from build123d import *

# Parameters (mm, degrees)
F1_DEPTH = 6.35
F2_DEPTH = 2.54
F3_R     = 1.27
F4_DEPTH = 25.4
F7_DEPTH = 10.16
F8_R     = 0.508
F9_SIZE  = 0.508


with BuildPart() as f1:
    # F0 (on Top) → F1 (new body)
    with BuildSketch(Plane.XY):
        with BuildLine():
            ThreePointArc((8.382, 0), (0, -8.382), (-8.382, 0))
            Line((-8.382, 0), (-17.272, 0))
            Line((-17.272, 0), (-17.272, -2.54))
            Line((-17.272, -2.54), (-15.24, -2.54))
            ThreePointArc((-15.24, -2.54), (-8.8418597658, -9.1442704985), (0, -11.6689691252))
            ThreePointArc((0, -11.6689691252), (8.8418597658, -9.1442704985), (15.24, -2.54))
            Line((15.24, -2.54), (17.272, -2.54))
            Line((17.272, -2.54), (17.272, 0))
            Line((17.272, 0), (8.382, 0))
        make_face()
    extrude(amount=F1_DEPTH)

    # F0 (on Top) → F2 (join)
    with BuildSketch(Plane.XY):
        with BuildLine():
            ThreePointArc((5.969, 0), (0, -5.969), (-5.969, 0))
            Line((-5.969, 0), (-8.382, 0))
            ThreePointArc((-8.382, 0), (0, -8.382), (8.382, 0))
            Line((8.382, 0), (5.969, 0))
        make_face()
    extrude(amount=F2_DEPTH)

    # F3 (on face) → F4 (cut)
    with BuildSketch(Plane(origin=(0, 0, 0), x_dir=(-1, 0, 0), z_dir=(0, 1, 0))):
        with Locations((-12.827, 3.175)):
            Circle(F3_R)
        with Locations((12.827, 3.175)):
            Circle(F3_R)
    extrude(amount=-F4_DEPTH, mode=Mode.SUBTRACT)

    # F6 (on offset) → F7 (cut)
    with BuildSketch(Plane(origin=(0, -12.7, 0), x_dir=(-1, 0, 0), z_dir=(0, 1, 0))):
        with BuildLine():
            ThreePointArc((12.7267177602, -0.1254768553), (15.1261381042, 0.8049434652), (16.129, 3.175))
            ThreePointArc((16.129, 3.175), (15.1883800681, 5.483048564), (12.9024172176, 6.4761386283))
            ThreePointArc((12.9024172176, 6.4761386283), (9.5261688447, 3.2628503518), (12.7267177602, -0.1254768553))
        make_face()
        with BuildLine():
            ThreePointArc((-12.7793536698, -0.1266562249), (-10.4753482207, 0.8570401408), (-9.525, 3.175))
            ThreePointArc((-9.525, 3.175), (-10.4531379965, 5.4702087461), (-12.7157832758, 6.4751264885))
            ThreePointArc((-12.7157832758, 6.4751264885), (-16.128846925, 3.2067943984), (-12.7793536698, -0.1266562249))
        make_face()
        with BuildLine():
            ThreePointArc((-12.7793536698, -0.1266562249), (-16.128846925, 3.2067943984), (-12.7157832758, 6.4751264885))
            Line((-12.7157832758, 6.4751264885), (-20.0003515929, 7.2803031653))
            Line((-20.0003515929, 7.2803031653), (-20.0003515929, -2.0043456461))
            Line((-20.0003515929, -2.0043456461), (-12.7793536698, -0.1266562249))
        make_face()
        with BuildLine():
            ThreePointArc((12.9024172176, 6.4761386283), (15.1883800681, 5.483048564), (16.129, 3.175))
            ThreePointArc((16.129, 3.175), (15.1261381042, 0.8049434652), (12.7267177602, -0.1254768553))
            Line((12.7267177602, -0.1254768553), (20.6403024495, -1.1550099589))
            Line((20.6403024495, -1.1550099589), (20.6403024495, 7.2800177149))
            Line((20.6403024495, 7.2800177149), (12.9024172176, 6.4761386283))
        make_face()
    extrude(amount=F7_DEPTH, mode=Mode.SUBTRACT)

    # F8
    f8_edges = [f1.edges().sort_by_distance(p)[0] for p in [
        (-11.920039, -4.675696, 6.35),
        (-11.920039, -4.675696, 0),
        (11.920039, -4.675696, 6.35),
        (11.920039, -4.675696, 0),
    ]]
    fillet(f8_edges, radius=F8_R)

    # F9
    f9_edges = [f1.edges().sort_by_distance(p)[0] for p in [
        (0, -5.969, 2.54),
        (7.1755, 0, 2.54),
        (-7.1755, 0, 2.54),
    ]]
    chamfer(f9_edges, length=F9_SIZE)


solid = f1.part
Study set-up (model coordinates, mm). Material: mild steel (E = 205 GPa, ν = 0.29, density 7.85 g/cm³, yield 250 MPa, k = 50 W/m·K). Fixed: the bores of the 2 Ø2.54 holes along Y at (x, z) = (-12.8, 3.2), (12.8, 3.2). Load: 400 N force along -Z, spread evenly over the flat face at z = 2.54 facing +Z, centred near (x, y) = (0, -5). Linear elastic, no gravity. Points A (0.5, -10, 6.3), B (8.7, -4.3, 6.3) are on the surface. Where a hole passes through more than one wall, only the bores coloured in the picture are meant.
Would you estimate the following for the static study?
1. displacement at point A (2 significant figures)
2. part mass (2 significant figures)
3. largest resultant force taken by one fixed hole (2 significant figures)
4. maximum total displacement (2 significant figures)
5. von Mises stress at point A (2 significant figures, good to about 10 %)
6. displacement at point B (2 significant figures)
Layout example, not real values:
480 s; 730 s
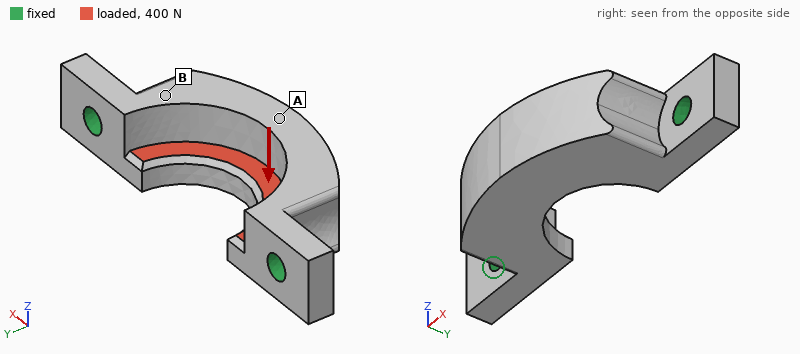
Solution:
10 µm; 7.8 g; 200 N; 12 µm; 23 MPa; 4.8 µm
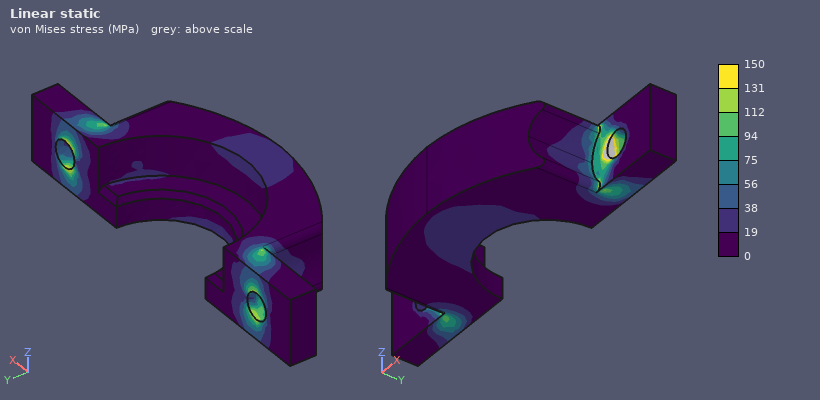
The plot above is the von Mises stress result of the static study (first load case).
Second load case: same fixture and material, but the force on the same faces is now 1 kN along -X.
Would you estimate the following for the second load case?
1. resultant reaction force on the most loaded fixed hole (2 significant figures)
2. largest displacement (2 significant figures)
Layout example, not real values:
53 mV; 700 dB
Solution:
520 N; 3.9 µm
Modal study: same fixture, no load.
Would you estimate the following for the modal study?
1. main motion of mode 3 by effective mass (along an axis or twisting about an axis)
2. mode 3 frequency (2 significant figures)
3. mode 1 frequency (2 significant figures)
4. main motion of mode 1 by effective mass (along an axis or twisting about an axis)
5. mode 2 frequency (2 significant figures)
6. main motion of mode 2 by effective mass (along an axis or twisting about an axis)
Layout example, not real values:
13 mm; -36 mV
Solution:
along Y; 36 kHz; 12 kHz; along Z; 29 kHz; along X
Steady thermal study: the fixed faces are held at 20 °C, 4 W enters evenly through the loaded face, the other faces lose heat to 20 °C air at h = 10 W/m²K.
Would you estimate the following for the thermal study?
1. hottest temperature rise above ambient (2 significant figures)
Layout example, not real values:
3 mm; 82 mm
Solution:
20 K
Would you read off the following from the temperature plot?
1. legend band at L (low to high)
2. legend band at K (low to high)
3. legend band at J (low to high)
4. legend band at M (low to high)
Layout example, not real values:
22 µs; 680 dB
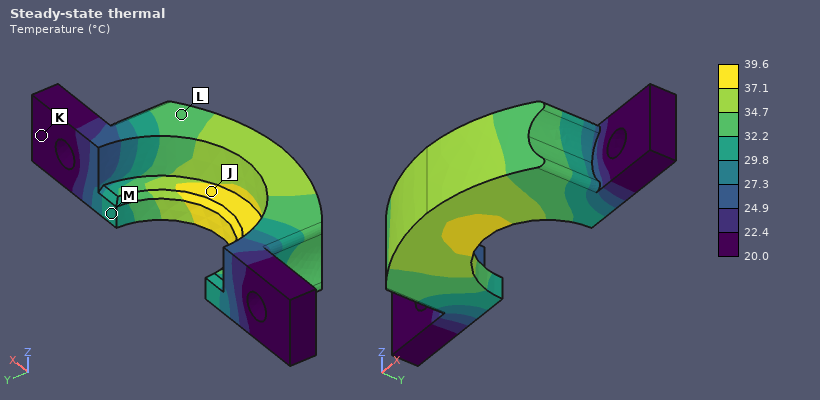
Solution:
32.2 to 34.7 °C; 20.0 to 22.4 °C; 37.1 to 39.6 °C; 29.8 to 32.2 °C
